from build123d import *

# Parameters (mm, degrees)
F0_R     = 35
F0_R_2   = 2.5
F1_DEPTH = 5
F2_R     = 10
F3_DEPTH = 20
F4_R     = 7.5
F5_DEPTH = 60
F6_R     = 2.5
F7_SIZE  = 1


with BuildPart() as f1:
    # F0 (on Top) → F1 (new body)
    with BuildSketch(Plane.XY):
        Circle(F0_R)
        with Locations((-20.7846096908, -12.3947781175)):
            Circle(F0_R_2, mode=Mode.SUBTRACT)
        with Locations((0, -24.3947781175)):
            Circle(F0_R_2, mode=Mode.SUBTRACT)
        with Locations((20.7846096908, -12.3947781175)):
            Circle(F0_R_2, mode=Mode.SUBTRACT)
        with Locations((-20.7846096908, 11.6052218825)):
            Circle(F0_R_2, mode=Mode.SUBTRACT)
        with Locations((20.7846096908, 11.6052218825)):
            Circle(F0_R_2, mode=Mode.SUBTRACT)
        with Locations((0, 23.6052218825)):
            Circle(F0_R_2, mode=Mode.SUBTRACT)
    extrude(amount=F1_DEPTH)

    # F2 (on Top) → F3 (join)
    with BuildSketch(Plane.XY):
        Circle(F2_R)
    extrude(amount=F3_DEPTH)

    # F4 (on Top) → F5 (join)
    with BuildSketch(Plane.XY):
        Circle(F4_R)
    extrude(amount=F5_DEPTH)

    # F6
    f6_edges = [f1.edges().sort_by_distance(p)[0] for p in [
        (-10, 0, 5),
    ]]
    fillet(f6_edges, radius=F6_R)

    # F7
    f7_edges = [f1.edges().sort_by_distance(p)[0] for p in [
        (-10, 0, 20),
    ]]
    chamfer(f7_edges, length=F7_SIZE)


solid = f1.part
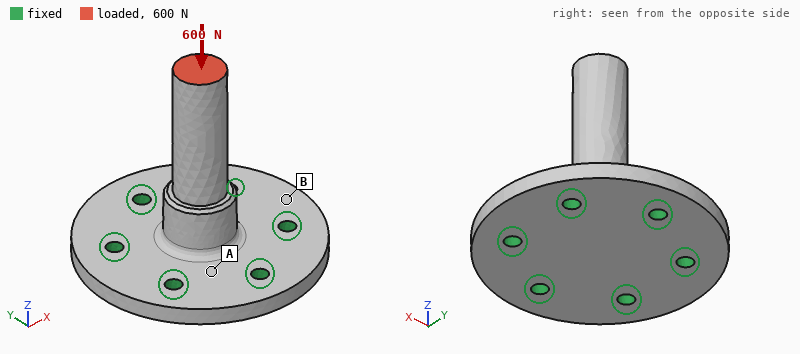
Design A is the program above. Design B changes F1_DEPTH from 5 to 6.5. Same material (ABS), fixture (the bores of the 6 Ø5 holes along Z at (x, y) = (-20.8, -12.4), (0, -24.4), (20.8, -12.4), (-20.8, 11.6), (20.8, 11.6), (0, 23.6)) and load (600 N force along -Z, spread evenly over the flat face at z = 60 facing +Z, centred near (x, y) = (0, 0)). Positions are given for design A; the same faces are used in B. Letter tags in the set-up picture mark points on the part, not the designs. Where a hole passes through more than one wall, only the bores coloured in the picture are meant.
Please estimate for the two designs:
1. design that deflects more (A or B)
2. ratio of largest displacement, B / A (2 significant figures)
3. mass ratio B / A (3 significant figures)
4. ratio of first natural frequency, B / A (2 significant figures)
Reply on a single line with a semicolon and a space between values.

A; 0.76; 1.17; 1.1
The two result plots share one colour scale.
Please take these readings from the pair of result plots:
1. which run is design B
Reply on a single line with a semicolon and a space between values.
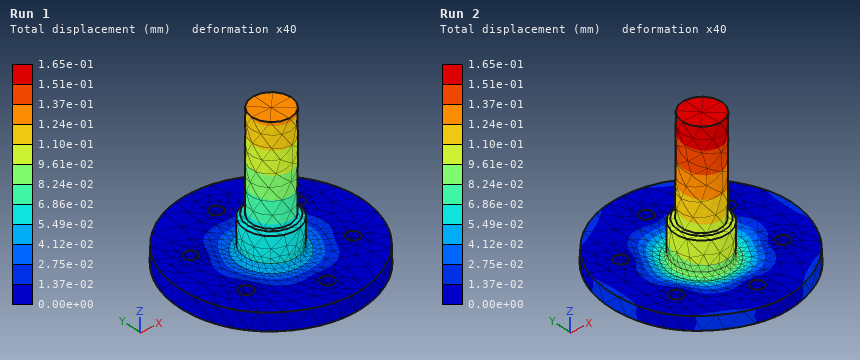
Run 1
